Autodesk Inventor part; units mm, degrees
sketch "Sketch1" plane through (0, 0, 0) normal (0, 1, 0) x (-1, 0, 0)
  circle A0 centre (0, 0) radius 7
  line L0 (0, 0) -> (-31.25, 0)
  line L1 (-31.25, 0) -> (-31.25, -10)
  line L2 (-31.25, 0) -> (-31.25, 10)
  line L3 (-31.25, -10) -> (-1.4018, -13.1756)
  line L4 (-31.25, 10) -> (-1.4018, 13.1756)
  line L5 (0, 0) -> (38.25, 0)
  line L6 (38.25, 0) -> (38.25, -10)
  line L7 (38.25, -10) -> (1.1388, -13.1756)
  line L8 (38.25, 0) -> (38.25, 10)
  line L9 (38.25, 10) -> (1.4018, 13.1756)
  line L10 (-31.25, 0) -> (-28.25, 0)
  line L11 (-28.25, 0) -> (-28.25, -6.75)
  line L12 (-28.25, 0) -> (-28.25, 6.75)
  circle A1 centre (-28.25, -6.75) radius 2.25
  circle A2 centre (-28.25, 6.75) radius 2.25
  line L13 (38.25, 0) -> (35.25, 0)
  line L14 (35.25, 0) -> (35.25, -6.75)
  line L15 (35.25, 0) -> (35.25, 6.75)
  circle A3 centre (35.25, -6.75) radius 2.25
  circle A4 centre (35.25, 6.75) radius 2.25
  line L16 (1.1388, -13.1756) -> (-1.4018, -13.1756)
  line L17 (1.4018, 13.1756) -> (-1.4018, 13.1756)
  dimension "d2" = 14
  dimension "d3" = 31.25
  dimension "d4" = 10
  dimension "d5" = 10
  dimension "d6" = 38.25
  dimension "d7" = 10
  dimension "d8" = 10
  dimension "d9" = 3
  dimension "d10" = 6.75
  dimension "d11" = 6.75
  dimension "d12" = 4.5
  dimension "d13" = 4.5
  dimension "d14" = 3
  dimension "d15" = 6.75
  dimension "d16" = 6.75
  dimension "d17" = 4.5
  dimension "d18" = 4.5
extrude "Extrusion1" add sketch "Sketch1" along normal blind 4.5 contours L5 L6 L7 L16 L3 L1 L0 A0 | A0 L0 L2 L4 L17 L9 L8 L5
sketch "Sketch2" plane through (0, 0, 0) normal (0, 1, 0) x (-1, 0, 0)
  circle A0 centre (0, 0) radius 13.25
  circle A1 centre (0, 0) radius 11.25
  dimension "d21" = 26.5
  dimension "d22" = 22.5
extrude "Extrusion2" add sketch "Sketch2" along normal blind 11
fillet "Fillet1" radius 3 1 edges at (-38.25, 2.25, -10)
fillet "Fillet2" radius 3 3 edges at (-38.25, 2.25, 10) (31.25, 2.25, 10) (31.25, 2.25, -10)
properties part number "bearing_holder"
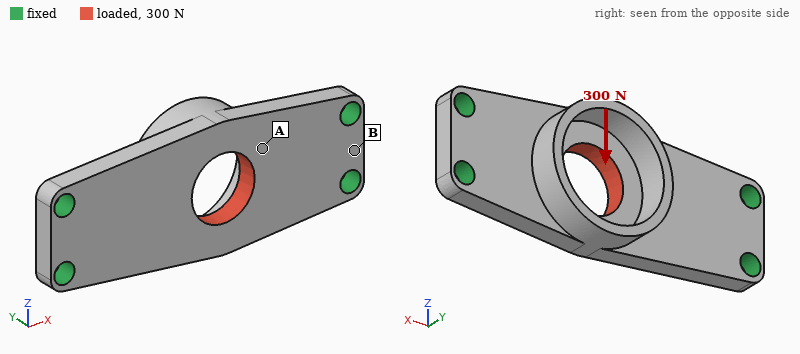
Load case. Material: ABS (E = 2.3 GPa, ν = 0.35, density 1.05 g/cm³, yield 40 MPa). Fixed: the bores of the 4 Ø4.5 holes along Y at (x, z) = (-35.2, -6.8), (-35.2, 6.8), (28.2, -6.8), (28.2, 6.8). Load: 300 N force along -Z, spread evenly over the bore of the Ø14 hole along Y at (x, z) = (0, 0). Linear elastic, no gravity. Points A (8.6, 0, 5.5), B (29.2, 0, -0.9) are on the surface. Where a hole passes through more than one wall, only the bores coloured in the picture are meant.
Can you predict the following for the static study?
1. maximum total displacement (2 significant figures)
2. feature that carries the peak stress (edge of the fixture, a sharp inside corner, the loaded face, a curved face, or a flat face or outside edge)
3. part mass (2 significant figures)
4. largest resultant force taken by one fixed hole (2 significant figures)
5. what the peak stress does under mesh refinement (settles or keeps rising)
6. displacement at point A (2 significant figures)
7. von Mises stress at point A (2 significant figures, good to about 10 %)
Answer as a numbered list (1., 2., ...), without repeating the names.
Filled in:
1. 87 µm
2. edge of the fixture
3. 7.6 g
4. 140 N
5. keeps rising
6. 59 µm
7. 2.7 MPa
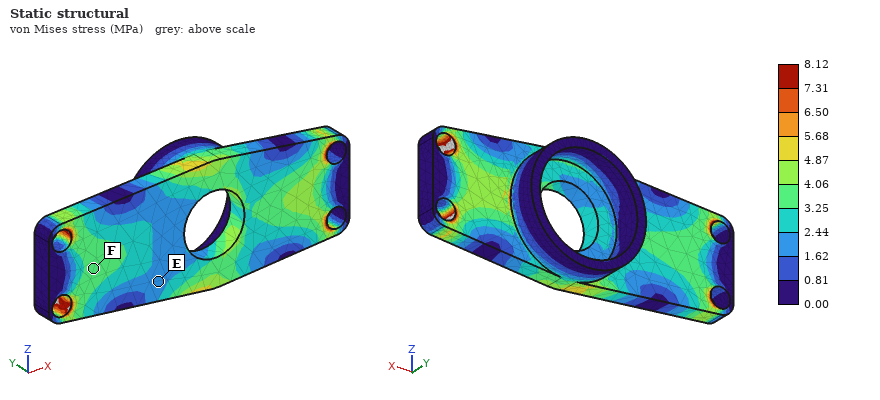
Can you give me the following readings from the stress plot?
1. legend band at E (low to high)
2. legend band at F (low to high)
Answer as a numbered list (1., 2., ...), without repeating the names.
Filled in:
1. 1.62 to 2.44 MPa
2. 3.25 to 4.06 MPa
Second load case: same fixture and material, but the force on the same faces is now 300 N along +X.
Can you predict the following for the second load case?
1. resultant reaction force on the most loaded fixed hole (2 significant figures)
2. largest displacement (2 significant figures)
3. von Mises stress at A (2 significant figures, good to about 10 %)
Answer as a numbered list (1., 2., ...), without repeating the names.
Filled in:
1. 82 N
2. 20 µm
3. 2.0 MPa
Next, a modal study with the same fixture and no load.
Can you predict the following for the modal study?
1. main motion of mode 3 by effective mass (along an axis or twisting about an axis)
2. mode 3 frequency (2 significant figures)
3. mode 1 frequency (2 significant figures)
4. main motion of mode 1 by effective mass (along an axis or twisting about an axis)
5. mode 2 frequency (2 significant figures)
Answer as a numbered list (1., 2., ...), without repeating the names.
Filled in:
1. twisting about Z
2. 4300 Hz
3. 1700 Hz
4. along Y
5. 2400 Hz
